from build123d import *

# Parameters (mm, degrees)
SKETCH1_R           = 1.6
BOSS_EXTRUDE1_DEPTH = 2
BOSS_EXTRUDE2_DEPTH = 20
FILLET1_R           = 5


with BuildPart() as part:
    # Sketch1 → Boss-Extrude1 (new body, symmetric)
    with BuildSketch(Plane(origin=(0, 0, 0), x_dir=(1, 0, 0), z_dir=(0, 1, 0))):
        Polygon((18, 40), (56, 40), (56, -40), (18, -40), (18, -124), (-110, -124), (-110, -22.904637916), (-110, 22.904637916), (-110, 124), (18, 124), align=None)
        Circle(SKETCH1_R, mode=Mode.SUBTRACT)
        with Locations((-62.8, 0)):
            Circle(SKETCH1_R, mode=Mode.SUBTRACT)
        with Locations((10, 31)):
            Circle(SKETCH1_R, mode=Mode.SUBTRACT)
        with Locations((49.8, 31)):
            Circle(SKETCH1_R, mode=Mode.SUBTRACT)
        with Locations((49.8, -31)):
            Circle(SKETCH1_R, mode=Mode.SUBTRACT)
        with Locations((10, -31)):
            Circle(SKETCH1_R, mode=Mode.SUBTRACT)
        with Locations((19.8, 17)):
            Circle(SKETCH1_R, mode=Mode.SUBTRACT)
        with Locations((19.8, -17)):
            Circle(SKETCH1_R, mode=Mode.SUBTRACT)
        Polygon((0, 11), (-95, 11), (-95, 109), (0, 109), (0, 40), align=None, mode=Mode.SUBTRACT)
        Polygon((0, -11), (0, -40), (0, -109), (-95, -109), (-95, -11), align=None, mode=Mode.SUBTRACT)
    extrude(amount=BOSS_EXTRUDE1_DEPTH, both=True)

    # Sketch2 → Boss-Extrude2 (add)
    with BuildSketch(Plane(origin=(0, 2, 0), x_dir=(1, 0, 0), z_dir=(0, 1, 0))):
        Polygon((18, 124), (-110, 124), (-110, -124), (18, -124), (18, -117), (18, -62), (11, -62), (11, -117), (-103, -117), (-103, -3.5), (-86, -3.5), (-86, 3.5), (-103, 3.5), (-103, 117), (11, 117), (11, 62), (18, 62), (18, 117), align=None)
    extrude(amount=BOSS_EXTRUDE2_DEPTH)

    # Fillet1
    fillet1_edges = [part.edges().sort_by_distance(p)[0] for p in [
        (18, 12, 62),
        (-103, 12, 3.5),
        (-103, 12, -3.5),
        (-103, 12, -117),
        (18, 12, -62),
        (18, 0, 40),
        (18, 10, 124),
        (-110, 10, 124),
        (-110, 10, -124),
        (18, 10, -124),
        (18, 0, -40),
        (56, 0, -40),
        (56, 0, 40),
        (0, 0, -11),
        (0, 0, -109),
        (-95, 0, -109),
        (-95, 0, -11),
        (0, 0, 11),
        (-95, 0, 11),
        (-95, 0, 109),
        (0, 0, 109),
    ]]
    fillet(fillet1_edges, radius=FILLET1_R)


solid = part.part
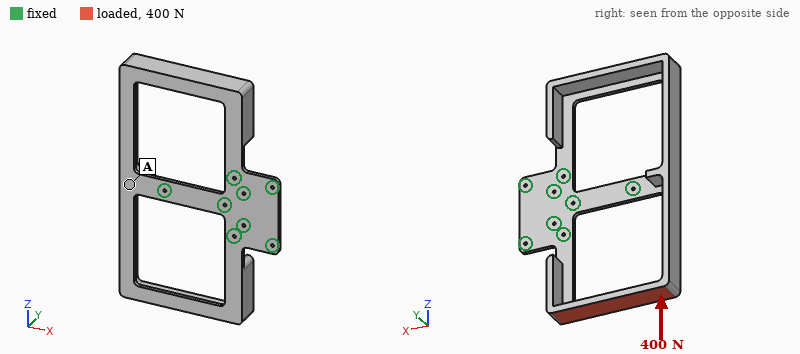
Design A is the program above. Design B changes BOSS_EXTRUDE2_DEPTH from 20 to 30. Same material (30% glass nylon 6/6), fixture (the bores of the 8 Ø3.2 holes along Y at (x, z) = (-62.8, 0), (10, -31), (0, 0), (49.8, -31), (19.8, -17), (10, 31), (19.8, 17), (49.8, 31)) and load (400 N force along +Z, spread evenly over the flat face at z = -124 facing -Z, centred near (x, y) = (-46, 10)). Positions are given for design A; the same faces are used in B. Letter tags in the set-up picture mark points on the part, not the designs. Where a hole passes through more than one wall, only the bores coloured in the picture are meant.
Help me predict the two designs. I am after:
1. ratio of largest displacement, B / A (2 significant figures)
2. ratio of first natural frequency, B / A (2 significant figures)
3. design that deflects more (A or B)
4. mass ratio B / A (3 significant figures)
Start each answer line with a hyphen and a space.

- 1.4
- 0.87
- B
- 1.29
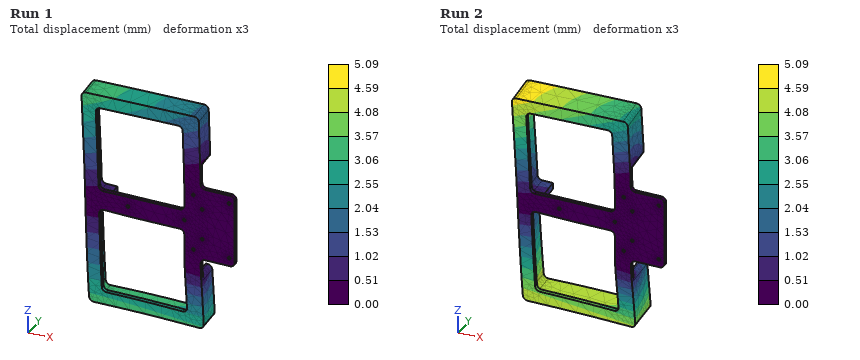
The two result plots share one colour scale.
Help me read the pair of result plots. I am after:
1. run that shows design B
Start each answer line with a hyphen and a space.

- Run 2
